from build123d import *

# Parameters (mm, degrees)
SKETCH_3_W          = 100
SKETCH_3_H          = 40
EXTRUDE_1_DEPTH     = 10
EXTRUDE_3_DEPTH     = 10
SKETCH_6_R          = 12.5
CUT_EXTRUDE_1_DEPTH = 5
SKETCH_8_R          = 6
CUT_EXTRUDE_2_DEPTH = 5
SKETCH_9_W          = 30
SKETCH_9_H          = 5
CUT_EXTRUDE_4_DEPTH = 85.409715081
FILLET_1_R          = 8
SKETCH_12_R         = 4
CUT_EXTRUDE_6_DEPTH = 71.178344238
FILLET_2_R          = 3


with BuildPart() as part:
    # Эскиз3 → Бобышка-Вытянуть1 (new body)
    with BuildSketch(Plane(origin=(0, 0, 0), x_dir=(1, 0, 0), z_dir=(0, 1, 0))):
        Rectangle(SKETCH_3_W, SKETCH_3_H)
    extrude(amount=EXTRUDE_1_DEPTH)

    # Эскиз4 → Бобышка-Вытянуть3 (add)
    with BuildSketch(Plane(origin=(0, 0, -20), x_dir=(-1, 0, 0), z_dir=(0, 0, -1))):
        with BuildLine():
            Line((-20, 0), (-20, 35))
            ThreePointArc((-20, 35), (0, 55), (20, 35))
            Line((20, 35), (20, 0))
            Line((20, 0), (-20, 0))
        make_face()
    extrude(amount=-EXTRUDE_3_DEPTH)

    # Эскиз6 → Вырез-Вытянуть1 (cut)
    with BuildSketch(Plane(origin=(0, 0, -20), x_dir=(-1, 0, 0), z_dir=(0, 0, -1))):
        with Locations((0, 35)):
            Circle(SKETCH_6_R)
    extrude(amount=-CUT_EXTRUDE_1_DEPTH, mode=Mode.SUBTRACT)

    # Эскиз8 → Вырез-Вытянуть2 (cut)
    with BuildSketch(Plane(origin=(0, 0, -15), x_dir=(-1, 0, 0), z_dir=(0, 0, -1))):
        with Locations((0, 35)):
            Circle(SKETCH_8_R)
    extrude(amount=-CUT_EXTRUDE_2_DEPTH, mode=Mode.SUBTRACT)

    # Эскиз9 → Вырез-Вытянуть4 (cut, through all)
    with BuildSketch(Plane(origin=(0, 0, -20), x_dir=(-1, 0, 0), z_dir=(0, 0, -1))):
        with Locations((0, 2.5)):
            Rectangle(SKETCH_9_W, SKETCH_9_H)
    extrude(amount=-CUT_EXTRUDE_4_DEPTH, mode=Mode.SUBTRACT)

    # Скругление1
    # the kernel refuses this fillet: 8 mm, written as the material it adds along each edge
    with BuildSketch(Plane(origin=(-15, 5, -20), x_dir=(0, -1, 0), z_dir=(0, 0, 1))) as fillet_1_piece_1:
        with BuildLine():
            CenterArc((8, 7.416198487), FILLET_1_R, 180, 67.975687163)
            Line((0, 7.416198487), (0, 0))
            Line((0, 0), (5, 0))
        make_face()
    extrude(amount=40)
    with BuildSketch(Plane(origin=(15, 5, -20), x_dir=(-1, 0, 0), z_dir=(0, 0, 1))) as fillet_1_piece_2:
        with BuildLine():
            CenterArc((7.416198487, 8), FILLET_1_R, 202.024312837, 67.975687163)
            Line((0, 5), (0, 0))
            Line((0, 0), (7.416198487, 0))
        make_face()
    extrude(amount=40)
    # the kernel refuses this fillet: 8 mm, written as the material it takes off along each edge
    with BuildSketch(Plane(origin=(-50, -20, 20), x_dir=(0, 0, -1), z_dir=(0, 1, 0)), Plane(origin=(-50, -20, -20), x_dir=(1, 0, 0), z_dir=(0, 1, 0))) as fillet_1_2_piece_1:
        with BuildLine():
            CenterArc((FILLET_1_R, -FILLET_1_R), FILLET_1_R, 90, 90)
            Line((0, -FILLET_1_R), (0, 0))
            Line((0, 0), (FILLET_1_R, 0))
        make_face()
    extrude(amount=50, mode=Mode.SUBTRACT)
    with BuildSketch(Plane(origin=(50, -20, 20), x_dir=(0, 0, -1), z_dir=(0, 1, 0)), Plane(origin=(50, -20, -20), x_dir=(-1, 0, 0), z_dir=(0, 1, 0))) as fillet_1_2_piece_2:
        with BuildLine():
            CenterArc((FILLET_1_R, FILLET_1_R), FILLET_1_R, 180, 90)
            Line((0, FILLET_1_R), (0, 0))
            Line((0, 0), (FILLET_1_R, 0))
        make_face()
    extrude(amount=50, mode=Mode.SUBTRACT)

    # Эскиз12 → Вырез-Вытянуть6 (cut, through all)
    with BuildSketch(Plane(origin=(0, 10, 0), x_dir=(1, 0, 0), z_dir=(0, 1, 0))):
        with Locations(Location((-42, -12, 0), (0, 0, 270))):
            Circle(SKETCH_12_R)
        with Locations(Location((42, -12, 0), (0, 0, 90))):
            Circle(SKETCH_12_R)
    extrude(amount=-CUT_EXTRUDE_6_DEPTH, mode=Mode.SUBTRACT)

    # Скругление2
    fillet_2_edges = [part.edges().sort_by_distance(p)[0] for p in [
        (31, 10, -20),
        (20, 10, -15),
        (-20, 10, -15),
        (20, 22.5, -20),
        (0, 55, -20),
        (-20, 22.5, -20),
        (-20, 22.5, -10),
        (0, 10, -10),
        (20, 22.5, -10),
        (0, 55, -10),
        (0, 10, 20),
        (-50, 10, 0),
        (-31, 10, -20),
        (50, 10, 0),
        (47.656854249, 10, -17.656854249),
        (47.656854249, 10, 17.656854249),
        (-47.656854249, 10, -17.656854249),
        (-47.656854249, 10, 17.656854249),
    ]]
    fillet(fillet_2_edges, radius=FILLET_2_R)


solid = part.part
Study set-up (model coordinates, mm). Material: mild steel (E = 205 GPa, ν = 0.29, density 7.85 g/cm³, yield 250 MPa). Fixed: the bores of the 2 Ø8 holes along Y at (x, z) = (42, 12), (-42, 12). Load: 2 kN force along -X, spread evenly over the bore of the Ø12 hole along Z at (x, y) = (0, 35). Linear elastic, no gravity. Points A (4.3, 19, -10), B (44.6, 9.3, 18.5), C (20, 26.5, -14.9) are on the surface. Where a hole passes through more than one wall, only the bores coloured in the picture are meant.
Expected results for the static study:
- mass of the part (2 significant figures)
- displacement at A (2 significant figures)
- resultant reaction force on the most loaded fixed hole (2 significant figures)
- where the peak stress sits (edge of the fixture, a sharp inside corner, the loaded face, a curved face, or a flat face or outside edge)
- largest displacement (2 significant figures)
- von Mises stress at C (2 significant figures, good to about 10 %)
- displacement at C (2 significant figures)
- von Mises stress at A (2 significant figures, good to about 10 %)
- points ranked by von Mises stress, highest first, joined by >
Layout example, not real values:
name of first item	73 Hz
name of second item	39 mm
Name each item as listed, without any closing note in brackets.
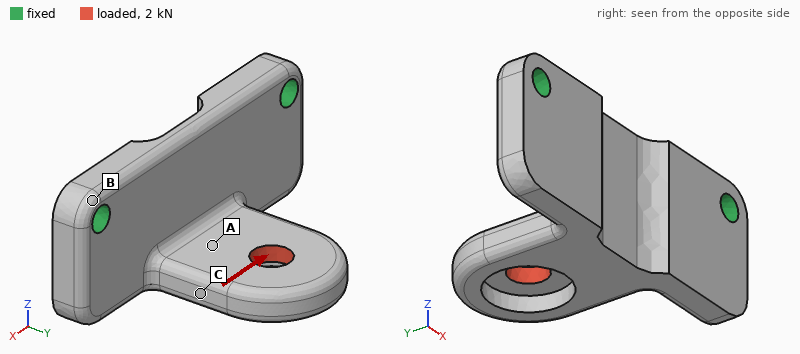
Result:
mass of the part	360 g
displacement at A	9.1 µm
resultant reaction force on the most loaded fixed hole	1.4 kN
where the peak stress sits	a curved face
largest displacement	33 µm
von Mises stress at C	13 MPa
displacement at C	19 µm
von Mises stress at A	23 MPa
points ranked by von Mises stress, highest first, joined by >	A > C > B
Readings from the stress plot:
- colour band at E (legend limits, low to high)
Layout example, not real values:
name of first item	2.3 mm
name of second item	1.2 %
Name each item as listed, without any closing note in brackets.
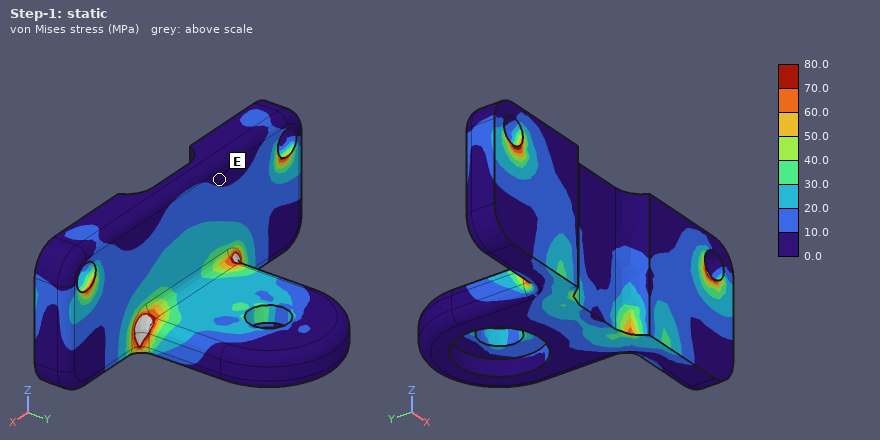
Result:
colour band at E	0.0 to 10.0 MPa
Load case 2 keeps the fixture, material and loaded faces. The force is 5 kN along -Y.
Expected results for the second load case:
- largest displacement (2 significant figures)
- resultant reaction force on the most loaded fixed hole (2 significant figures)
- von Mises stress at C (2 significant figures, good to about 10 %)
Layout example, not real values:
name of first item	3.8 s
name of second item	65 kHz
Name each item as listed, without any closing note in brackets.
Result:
largest displacement	0.10 mm
resultant reaction force on the most loaded fixed hole	2.8 kN
von Mises stress at C	19 MPa
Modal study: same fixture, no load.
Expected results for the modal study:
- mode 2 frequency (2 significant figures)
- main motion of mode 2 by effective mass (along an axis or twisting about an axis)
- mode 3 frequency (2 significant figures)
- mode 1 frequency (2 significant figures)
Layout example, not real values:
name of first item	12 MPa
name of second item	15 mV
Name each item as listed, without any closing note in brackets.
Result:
mode 2 frequency	4300 Hz
main motion of mode 2 by effective mass	along Y
mode 3 frequency	4700 Hz
mode 1 frequency	2300 Hz
